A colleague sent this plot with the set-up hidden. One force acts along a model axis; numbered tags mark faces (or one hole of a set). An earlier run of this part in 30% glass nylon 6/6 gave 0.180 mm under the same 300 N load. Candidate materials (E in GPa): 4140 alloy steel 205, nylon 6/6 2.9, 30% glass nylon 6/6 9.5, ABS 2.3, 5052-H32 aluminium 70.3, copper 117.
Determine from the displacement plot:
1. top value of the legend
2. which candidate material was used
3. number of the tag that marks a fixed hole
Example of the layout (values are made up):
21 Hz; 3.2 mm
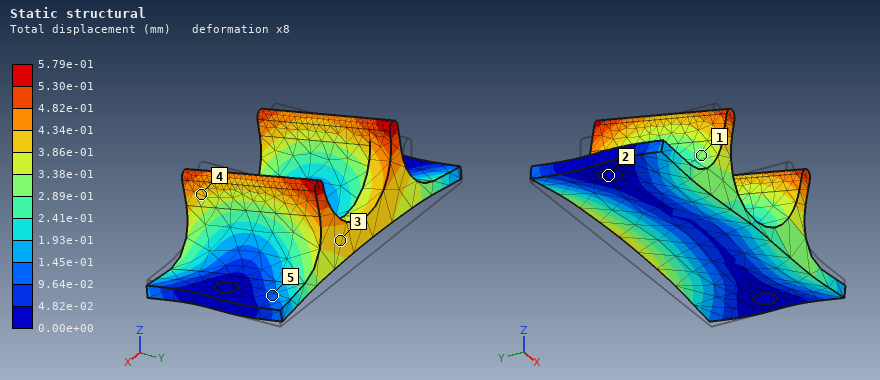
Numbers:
5.79e-01 mm; nylon 6/6; 2
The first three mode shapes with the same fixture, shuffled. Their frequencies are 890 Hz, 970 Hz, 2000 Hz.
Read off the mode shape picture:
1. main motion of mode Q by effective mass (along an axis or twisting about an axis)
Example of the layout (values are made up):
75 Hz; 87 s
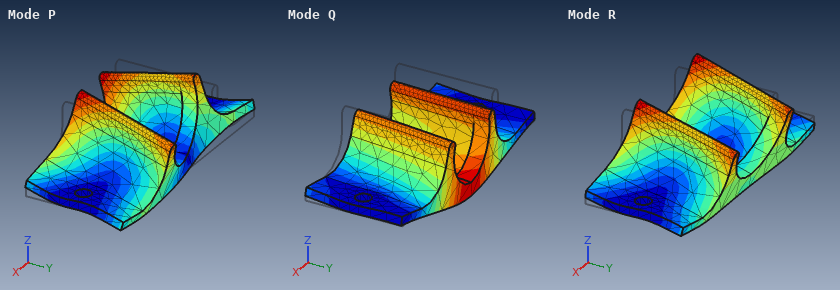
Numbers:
along Z
